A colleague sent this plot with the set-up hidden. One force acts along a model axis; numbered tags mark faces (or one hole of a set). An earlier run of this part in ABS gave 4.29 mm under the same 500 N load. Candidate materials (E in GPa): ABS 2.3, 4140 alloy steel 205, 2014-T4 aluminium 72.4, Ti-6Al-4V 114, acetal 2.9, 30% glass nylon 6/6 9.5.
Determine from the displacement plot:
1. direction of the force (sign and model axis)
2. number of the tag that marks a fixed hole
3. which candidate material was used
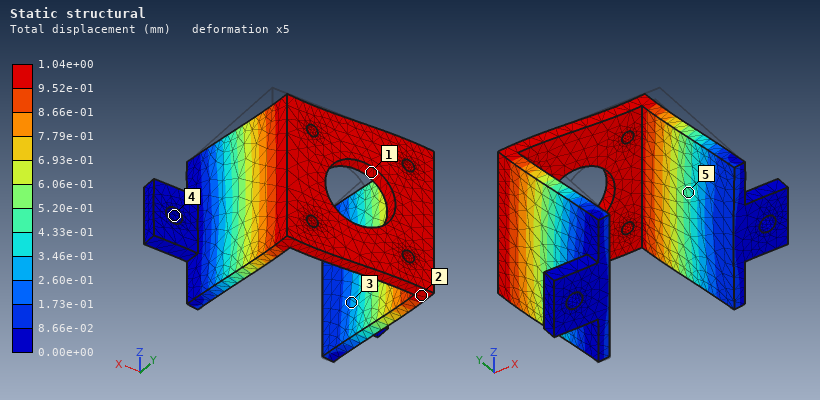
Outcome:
-X
4
30% glass nylon 6/6
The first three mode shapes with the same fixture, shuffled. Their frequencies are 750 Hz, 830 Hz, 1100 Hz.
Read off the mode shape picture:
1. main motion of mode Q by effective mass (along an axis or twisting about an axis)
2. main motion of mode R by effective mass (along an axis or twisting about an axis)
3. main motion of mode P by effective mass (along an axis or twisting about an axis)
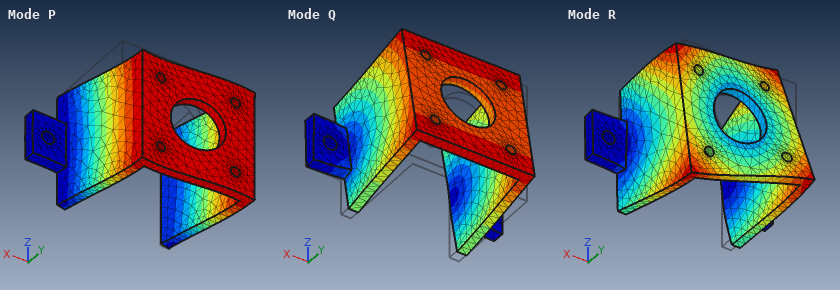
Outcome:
along Z
twisting about Y
along X
